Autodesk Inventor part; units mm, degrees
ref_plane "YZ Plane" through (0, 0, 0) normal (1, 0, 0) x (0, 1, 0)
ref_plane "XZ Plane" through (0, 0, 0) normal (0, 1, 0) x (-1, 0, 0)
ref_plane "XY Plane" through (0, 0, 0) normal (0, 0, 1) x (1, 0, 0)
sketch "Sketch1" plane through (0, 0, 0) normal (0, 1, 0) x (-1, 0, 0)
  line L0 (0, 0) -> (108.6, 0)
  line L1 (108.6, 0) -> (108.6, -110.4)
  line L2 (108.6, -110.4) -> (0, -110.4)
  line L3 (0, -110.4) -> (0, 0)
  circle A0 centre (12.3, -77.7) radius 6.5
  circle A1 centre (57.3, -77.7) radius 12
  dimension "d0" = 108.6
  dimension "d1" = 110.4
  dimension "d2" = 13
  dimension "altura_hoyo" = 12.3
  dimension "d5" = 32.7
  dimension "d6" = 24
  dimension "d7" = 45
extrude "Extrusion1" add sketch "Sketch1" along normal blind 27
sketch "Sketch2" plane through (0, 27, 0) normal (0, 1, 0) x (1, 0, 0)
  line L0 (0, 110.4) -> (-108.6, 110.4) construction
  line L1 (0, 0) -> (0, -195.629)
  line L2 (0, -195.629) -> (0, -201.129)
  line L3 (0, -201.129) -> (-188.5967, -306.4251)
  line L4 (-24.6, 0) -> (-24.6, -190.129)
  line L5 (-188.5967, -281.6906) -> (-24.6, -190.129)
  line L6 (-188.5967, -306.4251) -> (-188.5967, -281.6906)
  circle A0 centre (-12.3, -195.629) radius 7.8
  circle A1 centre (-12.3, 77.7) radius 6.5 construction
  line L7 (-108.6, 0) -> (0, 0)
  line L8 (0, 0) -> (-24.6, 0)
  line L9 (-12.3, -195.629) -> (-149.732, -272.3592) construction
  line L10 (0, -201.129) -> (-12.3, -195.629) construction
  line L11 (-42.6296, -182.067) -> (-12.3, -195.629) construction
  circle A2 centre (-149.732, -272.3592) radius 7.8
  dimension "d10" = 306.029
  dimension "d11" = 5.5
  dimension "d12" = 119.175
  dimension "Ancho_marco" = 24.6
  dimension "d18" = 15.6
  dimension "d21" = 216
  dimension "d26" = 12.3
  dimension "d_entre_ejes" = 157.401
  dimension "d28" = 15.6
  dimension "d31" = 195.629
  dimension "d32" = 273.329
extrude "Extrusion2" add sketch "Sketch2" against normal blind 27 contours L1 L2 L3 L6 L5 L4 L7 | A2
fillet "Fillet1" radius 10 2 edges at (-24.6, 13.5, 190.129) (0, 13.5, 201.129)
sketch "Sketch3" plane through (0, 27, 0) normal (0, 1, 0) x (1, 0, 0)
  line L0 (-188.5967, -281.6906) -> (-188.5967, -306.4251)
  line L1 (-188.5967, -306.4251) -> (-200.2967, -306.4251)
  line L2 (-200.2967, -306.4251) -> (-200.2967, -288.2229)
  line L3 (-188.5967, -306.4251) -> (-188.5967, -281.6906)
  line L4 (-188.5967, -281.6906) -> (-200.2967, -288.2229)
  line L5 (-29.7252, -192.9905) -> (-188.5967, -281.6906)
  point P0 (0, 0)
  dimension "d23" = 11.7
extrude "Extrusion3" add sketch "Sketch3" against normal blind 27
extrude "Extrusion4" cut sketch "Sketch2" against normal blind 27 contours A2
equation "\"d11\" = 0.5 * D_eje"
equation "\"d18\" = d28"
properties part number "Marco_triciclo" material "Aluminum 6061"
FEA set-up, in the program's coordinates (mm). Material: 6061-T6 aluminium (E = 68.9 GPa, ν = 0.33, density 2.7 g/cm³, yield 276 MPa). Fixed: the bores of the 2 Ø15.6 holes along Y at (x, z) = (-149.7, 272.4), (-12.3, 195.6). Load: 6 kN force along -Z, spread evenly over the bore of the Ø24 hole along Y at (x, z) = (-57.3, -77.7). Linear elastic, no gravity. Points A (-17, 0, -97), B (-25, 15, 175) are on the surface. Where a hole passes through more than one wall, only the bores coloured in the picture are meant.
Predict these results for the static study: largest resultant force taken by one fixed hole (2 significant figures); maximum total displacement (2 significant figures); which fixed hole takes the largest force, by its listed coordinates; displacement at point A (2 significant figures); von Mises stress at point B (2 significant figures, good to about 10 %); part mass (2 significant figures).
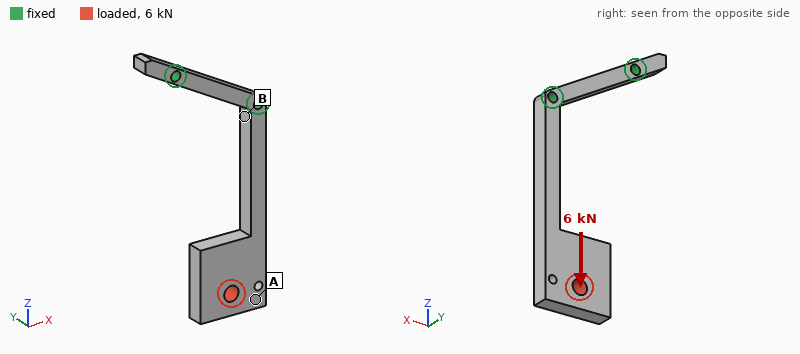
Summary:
5.7 kN
5.4 mm
(-12.3, 195.6)
4.5 mm
110 MPa
1.5 kg
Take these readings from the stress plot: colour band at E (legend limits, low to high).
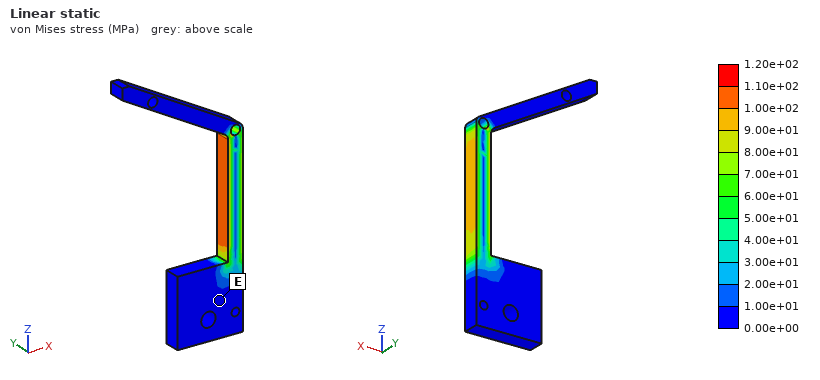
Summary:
0.00e+00 to 1.00e+01 MPa
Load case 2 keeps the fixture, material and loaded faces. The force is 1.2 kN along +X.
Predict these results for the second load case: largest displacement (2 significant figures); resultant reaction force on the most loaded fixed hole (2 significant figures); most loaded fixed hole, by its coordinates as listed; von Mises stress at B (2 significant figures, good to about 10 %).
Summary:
4.4 mm
1.0 kN
(-12.3, 195.6)
110 MPa
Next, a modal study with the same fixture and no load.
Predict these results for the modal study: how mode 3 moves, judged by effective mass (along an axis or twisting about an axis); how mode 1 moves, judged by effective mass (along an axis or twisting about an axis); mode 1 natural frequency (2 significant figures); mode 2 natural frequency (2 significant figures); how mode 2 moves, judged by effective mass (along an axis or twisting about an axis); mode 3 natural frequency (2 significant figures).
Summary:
twisting about Z
along X
110 Hz
120 Hz
along Y
480 Hz
